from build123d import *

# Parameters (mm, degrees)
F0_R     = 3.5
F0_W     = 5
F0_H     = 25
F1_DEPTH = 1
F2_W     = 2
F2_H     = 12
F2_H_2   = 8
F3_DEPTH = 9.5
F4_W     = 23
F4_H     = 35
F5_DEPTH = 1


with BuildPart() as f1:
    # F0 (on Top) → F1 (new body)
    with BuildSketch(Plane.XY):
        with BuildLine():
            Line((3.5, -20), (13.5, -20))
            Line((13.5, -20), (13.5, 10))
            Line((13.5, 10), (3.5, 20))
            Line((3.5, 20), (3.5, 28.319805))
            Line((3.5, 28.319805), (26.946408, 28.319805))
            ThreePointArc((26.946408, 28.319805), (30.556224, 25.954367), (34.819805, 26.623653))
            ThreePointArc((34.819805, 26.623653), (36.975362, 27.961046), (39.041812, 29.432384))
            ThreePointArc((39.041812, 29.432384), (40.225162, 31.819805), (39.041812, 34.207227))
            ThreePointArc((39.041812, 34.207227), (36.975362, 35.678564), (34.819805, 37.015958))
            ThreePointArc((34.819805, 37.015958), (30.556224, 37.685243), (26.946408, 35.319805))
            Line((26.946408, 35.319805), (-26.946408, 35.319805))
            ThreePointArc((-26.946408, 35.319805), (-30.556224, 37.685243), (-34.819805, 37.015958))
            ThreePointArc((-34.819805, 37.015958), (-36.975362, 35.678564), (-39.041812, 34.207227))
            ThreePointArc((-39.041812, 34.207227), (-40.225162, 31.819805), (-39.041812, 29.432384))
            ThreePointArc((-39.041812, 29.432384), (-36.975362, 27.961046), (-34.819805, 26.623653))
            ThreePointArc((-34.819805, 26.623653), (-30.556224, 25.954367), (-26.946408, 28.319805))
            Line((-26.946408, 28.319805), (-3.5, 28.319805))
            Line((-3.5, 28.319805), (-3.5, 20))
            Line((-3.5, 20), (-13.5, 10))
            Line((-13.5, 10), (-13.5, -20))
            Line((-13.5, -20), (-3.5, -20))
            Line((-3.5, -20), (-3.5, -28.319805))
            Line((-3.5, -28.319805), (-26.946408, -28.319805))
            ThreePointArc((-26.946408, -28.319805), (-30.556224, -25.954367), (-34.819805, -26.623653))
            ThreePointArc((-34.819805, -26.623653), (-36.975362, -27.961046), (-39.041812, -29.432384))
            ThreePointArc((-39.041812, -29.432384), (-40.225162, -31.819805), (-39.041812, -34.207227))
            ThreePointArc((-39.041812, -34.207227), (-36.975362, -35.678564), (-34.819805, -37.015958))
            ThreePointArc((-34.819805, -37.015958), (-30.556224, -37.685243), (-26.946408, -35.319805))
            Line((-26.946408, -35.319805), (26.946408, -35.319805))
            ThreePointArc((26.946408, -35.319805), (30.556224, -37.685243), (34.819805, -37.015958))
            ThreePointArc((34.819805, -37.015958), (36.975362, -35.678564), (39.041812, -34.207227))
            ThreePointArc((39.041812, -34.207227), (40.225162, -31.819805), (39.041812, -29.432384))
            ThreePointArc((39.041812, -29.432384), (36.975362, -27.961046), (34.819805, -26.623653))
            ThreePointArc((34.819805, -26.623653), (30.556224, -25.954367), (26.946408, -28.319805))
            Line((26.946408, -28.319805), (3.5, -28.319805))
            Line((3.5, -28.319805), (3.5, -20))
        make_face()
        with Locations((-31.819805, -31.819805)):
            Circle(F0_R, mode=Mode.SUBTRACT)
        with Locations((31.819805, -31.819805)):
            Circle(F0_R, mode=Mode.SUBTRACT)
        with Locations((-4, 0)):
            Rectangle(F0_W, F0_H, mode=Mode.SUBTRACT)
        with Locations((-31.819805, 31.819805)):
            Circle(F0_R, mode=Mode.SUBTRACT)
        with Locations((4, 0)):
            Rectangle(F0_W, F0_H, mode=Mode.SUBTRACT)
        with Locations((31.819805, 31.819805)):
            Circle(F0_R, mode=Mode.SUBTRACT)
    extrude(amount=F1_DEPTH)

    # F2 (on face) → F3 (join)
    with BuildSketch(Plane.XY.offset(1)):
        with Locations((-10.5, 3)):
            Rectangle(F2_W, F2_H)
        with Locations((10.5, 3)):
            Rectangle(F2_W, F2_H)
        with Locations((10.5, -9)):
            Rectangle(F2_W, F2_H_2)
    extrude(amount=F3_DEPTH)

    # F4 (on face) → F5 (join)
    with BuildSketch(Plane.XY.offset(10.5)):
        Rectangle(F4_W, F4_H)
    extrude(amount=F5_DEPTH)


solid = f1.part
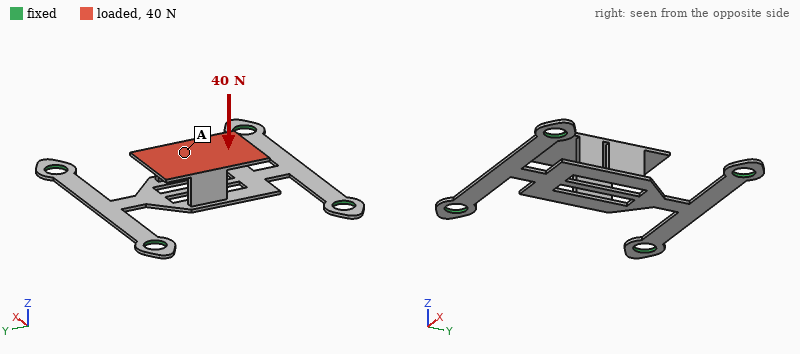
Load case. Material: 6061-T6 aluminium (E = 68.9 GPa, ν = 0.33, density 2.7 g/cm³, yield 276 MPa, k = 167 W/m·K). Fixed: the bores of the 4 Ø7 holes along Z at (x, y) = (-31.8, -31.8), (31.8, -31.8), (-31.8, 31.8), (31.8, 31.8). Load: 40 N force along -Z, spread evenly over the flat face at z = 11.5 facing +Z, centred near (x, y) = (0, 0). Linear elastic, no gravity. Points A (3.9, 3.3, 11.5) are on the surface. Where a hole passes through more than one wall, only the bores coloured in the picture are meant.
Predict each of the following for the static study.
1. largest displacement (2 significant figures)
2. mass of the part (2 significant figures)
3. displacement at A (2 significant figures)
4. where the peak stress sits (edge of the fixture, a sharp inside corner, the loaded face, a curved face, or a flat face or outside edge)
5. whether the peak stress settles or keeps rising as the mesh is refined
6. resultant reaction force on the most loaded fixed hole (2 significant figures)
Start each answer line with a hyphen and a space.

- 1.3 mm
- 9.0 g
- 1.2 mm
- a sharp inside corner
- keeps rising
- 11 N
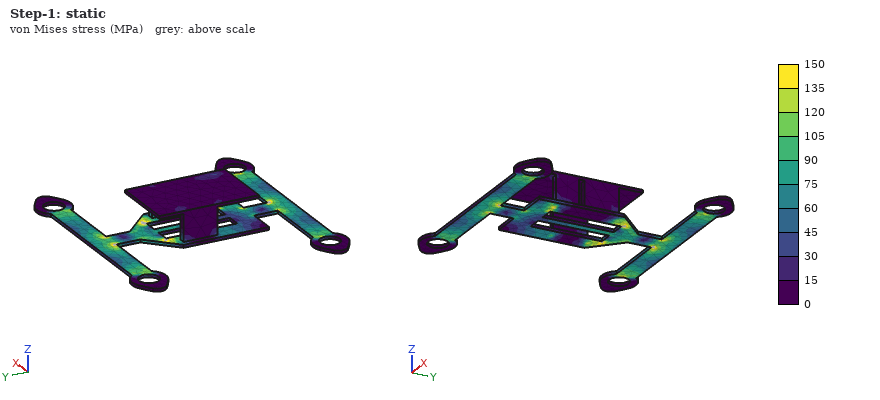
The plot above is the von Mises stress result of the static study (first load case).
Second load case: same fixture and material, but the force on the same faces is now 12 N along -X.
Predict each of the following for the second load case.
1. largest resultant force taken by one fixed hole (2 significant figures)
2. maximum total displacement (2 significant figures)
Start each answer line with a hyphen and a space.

- 3.7 N
- 0.37 mm
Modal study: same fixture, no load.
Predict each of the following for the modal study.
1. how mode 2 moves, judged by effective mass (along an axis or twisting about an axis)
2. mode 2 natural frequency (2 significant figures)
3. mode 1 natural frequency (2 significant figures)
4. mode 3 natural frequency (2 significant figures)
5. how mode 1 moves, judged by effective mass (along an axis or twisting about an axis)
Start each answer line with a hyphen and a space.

- along X
- 470 Hz
- 390 Hz
- 820 Hz
- along Z
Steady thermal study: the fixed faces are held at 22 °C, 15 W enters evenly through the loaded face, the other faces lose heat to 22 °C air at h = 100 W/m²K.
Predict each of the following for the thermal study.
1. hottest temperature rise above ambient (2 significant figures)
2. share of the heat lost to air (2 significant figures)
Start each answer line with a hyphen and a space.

- 56 K
- 90 %
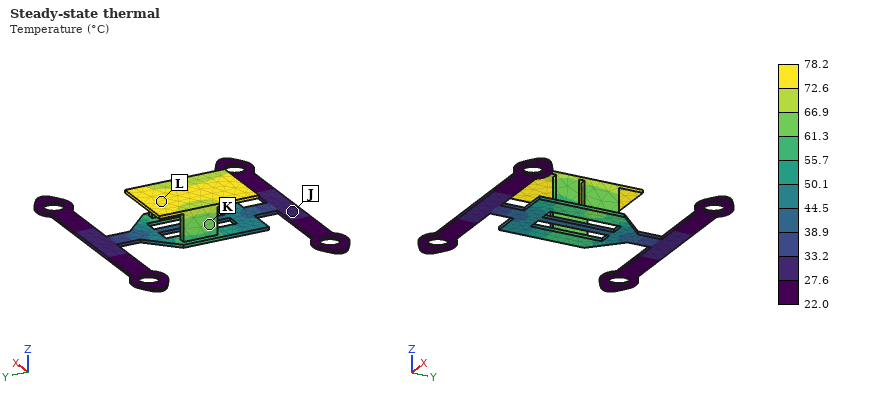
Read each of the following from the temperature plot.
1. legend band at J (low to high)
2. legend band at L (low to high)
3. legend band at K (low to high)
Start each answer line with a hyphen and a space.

- 27.6 to 33.2 °C
- 72.6 to 78.2 °C
- 61.3 to 66.9 °C
